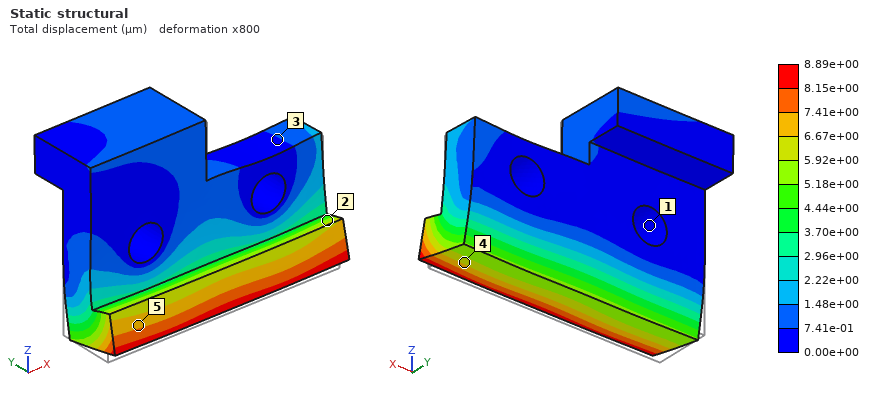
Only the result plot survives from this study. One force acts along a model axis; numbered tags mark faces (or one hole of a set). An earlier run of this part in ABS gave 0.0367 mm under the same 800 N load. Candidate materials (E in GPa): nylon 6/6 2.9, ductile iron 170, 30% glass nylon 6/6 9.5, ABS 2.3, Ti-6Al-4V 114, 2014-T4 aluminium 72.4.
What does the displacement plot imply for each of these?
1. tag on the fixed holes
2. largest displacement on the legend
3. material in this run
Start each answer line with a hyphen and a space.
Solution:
- 1
- 8.89e+00 µm
- 30% glass nylon 6/6
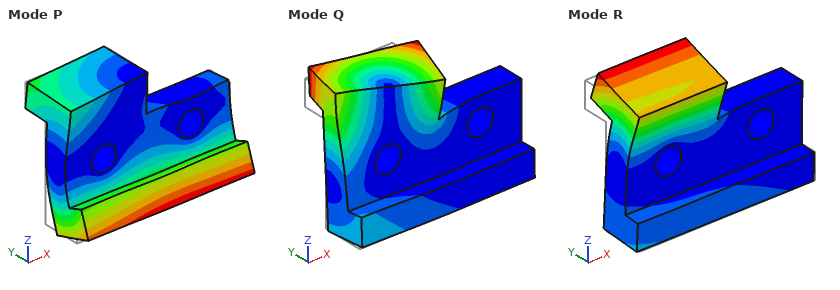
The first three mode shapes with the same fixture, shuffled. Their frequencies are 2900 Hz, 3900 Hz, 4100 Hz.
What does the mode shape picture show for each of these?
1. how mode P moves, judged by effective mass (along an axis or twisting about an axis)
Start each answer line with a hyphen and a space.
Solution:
- along Y
